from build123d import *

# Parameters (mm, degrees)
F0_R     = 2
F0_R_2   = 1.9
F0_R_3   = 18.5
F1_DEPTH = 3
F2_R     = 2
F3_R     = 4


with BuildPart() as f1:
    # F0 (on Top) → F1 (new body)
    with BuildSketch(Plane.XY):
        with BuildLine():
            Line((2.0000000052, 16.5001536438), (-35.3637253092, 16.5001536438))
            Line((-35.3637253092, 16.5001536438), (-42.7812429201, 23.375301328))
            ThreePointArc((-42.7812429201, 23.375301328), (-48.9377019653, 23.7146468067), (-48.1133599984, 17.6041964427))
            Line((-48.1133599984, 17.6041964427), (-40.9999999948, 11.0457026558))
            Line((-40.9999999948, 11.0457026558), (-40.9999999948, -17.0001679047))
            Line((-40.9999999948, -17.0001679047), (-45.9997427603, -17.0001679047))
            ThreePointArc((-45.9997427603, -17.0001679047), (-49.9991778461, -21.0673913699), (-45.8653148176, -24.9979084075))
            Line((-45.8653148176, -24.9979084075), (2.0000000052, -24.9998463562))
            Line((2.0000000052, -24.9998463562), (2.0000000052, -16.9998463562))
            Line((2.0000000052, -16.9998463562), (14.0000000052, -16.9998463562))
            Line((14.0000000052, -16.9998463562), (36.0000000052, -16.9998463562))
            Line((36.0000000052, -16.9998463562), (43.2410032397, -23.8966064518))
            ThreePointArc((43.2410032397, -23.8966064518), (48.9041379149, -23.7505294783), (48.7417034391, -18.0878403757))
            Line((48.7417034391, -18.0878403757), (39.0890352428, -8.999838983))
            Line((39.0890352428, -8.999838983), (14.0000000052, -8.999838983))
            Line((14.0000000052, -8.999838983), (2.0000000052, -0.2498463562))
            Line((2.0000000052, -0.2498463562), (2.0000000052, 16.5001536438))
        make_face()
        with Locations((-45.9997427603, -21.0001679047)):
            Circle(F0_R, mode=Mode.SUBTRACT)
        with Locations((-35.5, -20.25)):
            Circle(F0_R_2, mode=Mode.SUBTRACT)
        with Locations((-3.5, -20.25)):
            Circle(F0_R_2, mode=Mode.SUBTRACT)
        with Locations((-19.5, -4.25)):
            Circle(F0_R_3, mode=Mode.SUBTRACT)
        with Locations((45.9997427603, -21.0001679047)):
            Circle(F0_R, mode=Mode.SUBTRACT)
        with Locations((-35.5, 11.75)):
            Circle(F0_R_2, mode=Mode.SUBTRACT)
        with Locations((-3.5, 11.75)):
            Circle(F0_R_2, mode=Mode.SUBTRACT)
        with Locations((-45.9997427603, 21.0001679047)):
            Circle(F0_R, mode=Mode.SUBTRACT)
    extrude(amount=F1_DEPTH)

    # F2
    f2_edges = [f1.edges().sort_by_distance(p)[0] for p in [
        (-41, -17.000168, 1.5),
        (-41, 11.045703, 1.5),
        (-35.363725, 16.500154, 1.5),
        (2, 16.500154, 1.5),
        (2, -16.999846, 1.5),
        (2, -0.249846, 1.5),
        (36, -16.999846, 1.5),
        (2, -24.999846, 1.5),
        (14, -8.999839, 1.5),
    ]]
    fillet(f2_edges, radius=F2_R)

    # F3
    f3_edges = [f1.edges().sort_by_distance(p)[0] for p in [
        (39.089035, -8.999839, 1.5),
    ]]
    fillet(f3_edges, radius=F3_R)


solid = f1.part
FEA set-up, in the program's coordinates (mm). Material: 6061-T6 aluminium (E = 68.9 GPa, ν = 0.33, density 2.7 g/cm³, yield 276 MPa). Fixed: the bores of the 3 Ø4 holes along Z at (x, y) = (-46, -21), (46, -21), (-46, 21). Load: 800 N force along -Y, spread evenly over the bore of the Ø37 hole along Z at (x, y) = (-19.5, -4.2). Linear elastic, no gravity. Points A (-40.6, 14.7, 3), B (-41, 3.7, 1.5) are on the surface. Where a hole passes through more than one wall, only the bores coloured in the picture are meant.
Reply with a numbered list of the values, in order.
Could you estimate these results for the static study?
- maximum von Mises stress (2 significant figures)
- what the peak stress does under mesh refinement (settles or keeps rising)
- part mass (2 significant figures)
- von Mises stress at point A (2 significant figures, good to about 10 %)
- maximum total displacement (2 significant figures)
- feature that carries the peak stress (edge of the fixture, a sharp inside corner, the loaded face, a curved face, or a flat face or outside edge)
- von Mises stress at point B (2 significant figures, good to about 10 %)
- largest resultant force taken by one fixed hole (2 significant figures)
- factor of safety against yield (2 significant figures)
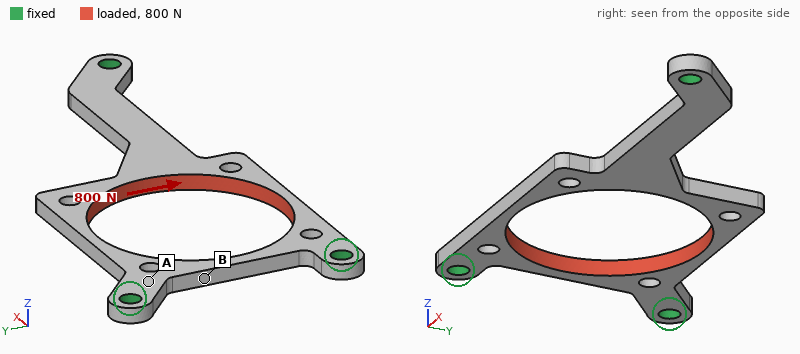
1. 250 MPa
2. settles
3. 10 g
4. 23 MPa
5. 0.26 mm
6. a curved face
7. 90 MPa
8. 310 N
9. 1.1
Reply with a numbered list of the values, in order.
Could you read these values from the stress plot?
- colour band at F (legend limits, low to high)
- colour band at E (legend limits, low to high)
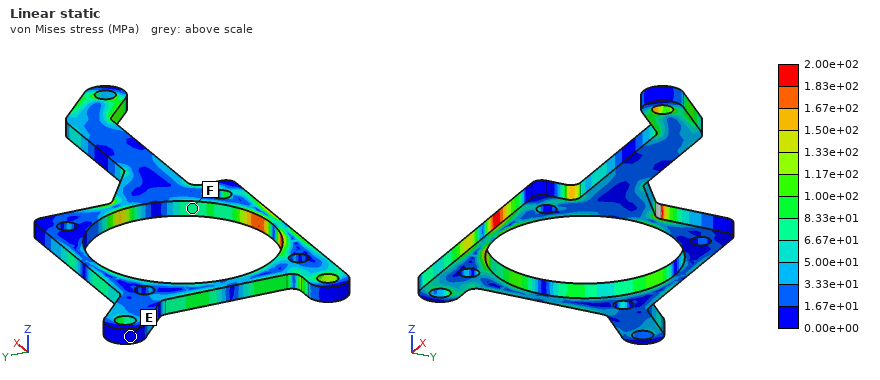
1. 6.67e+01 to 8.33e+01 MPa
2. 0.00e+00 to 1.67e+01 MPa
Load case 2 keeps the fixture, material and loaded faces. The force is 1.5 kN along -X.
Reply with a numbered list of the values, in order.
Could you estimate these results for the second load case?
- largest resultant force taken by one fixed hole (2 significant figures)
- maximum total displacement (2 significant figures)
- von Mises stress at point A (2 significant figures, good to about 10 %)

1. 640 N
2. 70 µm
3. 33 MPa
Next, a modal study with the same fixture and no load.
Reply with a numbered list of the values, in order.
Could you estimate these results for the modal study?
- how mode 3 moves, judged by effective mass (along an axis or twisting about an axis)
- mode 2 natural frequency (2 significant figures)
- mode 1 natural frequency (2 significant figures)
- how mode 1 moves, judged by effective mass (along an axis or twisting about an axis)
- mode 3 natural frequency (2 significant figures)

1. along Y
2. 2400 Hz
3. 1400 Hz
4. along Z
5. 3300 Hz
